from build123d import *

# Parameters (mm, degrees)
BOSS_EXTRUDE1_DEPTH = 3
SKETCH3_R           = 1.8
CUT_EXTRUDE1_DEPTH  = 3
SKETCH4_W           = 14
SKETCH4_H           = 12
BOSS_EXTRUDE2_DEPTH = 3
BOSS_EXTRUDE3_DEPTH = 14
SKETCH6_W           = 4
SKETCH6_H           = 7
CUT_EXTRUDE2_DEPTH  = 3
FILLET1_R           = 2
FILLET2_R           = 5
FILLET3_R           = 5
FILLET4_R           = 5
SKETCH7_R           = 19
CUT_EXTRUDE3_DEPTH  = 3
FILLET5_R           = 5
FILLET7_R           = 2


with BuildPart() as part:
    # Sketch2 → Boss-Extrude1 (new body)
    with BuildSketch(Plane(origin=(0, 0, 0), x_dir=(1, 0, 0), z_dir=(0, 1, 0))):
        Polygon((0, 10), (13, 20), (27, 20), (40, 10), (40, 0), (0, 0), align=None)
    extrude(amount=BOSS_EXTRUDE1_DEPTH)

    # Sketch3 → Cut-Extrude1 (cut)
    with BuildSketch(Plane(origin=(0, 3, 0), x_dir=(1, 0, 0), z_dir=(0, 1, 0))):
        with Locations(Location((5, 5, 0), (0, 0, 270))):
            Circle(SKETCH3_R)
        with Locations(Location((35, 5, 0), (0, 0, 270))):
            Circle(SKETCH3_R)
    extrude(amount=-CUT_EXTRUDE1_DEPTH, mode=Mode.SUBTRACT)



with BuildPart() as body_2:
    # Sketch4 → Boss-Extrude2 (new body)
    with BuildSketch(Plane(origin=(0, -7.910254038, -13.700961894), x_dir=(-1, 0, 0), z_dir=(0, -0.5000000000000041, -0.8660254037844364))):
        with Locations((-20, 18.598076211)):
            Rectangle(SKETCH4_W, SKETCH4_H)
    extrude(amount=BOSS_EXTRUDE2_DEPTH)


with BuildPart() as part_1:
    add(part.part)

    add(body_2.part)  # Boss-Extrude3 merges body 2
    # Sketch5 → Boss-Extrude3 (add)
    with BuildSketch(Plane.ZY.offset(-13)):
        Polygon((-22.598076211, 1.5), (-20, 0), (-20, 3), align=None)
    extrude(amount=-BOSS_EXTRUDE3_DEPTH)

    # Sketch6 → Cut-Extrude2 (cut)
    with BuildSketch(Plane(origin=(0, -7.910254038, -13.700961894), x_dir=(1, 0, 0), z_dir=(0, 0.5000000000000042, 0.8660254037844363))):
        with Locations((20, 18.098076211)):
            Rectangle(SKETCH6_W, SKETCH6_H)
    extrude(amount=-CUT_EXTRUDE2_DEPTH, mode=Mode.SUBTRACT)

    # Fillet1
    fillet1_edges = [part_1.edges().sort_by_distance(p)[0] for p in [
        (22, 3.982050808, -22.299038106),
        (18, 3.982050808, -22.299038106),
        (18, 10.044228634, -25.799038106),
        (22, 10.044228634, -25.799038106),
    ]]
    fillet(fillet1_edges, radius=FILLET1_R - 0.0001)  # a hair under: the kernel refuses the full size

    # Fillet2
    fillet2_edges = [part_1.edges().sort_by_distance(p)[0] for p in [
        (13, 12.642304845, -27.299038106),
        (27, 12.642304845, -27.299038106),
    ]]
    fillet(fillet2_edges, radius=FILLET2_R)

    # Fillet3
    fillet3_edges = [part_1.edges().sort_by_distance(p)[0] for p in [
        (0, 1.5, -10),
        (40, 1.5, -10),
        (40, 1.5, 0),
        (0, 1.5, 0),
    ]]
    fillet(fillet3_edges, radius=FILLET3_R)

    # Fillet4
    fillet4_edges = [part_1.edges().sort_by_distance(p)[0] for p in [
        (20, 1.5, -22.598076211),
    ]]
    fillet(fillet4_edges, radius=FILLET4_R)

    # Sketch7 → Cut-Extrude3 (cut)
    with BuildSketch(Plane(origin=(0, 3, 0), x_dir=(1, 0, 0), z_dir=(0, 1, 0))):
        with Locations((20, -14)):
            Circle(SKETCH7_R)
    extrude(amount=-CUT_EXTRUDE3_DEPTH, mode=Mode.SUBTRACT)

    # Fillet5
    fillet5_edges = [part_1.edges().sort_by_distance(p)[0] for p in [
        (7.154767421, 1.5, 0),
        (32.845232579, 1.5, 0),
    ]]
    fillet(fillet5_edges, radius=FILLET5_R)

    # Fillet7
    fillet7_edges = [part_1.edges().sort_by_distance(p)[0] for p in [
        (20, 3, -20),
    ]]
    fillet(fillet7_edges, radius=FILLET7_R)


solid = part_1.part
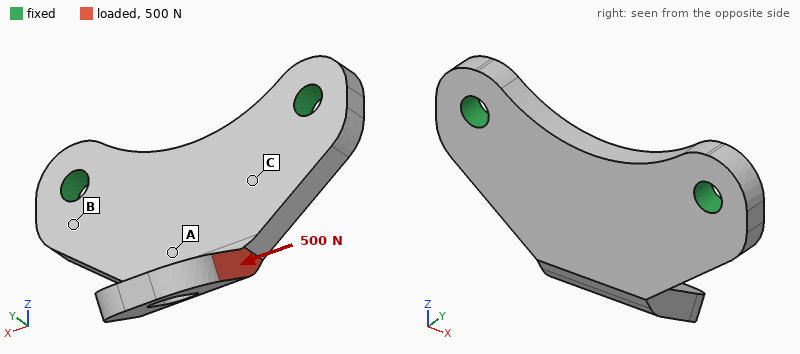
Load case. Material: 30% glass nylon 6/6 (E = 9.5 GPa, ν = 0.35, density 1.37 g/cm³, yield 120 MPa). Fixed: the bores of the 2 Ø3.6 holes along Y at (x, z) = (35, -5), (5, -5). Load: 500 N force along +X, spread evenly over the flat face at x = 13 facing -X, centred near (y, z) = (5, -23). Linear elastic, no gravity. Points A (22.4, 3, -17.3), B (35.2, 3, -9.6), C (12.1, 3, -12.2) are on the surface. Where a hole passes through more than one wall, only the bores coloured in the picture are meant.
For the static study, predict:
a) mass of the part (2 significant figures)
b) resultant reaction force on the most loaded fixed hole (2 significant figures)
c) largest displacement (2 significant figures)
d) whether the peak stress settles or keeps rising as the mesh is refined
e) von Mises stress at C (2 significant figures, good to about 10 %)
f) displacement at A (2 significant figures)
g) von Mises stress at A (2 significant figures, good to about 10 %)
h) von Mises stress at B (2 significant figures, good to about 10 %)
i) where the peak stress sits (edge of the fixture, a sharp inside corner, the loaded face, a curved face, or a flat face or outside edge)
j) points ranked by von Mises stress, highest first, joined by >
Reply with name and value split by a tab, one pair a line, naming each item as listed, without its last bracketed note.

mass of the part	2.9 g
resultant reaction force on the most loaded fixed hole	390 N
largest displacement	0.33 mm
whether the peak stress settles or keeps rising as the mesh is refined	keeps rising
von Mises stress at C	26 MPa
displacement at A	0.060 mm
von Mises stress at A	44 MPa
von Mises stress at B	8.8 MPa
where the peak stress sits	a sharp inside corner
points ranked by von Mises stress, highest first, joined by >	A > C > B
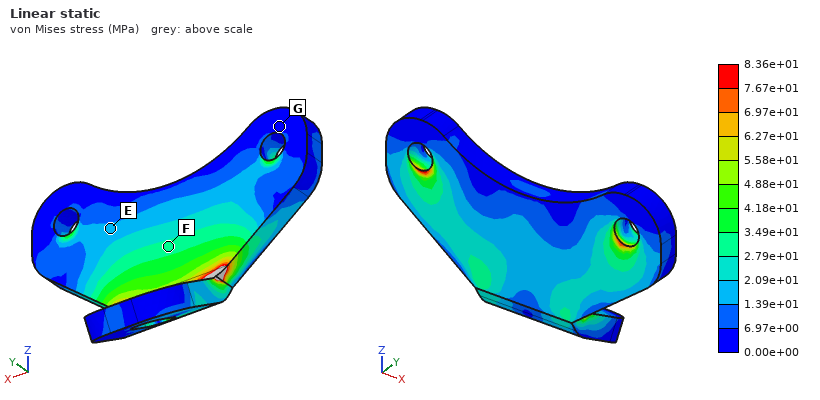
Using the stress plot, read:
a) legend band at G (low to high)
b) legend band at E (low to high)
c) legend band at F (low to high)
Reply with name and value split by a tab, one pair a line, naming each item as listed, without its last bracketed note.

legend band at G	0.00e+00 to 6.97e+00 MPa
legend band at E	1.39e+01 to 2.09e+01 MPa
legend band at F	2.79e+01 to 3.49e+01 MPa
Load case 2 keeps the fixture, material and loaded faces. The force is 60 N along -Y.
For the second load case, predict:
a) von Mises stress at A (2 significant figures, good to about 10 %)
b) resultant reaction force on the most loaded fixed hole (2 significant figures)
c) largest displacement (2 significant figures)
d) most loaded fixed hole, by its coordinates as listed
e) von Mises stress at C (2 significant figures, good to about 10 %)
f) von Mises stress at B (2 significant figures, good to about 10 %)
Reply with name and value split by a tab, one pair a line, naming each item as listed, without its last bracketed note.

von Mises stress at A	14 MPa
resultant reaction force on the most loaded fixed hole	47 N
largest displacement	0.49 mm
most loaded fixed hole, by its coordinates as listed	(5, -5)
von Mises stress at C	19 MPa
von Mises stress at B	17 MPa
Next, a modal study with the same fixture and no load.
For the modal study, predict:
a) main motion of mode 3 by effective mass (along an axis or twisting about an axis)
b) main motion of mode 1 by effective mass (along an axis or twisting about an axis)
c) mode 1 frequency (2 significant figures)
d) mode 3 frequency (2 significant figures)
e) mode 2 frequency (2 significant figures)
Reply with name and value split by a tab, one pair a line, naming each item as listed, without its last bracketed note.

main motion of mode 3 by effective mass	along Y
main motion of mode 1 by effective mass	along Y
mode 1 frequency	2200 Hz
mode 3 frequency	6700 Hz
mode 2 frequency	6200 Hz
